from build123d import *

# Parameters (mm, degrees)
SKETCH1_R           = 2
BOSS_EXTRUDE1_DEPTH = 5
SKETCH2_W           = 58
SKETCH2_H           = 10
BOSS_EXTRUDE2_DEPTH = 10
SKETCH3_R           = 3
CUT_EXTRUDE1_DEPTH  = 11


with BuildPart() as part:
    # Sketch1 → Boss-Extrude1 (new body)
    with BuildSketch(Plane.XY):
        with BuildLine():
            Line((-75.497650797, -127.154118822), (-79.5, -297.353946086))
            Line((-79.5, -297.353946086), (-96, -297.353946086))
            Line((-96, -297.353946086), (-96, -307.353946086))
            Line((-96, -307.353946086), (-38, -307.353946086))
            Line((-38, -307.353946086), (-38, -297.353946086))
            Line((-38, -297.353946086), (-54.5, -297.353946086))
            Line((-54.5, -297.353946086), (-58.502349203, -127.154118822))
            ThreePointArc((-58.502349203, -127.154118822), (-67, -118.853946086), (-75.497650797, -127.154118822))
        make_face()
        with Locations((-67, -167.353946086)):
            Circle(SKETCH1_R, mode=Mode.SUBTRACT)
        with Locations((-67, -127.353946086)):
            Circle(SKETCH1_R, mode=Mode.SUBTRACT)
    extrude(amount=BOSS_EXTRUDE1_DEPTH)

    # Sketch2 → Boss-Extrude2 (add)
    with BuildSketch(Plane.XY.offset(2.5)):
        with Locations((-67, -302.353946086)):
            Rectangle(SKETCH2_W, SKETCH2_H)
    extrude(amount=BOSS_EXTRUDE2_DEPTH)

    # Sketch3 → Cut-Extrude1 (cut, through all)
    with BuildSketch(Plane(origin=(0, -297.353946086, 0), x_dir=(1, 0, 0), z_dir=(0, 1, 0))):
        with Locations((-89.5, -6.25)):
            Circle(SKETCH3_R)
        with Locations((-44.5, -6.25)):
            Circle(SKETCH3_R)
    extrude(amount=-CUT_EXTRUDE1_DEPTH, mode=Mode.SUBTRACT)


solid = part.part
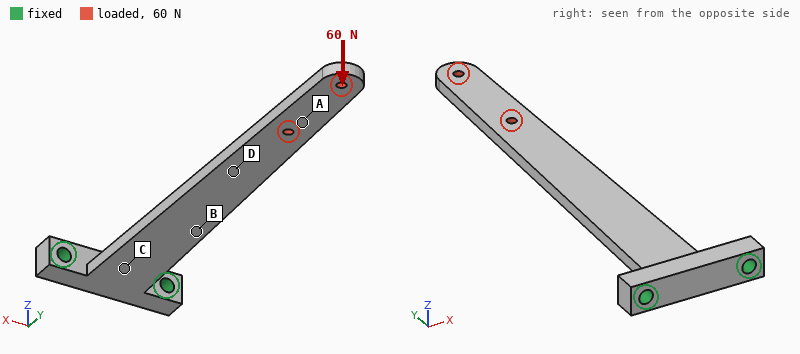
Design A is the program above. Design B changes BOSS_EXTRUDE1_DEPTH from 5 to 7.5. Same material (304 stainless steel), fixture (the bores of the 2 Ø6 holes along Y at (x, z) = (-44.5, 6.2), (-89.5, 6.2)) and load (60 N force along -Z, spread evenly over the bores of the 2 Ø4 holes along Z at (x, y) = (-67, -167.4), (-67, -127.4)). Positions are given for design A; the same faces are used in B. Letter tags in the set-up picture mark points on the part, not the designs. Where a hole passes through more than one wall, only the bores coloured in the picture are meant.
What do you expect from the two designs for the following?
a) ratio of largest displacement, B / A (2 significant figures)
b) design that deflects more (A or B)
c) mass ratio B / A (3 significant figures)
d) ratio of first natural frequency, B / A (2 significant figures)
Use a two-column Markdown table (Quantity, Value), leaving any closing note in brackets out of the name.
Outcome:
| Quantity | Value |
|---|---|
| ratio of largest displacement, B / A | 0.32 |
| design that deflects more | A |
| mass ratio B / A | 1.37 |
| ratio of first natural frequency, B / A | 1.4 |
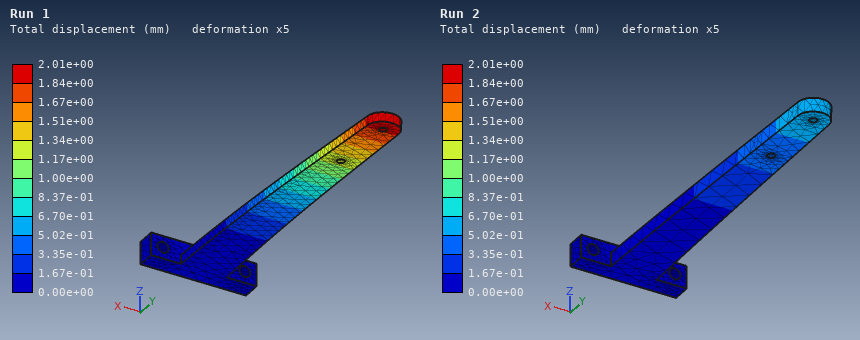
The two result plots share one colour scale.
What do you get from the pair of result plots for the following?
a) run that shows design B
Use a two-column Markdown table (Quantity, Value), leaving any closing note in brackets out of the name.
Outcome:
| Quantity | Value |
|---|---|
| run that shows design B | Run 2 |
